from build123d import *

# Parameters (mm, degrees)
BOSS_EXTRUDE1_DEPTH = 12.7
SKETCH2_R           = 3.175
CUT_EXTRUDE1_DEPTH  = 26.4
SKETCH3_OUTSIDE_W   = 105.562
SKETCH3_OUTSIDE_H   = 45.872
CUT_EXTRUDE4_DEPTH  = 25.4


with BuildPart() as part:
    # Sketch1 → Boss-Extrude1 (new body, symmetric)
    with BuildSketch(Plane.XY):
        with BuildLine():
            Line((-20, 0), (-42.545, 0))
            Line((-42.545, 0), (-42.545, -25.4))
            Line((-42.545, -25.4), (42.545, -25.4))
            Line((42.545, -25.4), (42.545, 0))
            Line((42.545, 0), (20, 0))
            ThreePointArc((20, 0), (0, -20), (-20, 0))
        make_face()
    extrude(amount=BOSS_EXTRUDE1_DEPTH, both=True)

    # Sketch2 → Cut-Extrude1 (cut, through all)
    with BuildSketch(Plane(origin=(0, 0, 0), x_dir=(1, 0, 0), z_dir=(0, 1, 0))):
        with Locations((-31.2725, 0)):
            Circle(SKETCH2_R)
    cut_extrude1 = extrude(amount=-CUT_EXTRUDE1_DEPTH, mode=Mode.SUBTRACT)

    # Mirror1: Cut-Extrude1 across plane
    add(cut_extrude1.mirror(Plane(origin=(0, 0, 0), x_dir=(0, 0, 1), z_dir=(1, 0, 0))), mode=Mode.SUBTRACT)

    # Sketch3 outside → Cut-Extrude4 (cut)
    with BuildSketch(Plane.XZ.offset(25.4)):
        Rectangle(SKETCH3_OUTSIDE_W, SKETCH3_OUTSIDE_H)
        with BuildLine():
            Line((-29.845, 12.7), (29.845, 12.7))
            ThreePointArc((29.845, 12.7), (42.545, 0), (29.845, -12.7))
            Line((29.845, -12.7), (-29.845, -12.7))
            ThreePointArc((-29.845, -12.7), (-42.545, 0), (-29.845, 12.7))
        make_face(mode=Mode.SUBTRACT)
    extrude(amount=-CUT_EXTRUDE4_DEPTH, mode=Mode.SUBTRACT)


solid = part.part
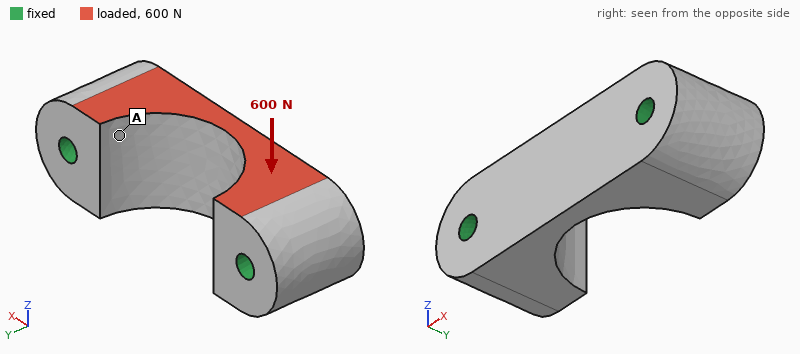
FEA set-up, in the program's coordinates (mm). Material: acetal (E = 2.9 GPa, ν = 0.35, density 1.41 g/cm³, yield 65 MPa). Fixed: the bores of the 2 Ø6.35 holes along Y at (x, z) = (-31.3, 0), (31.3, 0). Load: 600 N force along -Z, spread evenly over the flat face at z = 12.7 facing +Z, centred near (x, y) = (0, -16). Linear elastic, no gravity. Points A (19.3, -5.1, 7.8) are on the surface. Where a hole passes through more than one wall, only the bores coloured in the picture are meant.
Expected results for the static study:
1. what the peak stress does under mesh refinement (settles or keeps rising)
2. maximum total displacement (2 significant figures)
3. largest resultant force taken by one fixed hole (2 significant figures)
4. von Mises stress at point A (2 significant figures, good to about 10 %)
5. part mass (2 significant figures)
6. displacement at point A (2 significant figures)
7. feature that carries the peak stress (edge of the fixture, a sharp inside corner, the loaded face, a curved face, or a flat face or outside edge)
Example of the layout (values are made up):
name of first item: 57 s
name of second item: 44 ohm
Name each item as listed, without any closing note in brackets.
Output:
what the peak stress does under mesh refinement: keeps rising
maximum total displacement: 31 µm
largest resultant force taken by one fixed hole: 300 N
von Mises stress at point A: 0.77 MPa
part mass: 48 g
displacement at point A: 12 µm
feature that carries the peak stress: edge of the fixture
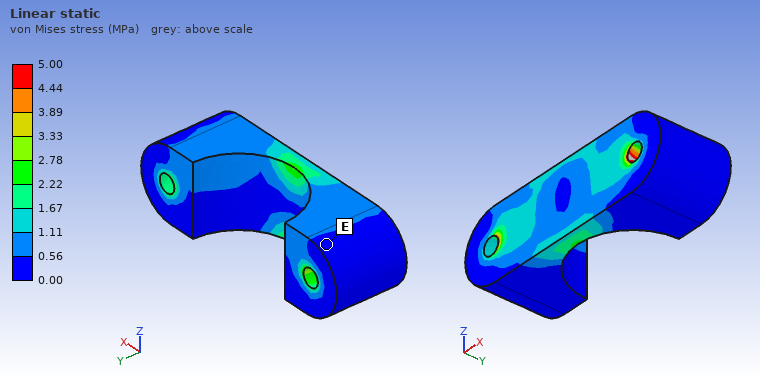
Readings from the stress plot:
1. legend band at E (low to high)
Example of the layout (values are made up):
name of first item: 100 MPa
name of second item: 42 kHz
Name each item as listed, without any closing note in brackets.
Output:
legend band at E: 0.00 to 0.56 MPa
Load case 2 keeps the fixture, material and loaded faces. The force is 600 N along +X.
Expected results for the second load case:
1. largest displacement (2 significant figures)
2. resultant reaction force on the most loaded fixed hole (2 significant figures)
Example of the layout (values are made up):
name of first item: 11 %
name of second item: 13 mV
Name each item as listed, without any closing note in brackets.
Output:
largest displacement: 14 µm
resultant reaction force on the most loaded fixed hole: 310 N
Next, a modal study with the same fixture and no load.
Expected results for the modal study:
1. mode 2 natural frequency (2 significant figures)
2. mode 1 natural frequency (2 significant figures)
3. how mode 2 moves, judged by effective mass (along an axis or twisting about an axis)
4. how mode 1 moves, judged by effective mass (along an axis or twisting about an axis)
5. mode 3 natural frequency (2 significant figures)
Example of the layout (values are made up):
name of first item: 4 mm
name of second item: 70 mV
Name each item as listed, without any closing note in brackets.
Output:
mode 2 natural frequency: 6600 Hz
mode 1 natural frequency: 4900 Hz
how mode 2 moves, judged by effective mass: along Y
how mode 1 moves, judged by effective mass: along Z
mode 3 natural frequency: 8900 Hz
